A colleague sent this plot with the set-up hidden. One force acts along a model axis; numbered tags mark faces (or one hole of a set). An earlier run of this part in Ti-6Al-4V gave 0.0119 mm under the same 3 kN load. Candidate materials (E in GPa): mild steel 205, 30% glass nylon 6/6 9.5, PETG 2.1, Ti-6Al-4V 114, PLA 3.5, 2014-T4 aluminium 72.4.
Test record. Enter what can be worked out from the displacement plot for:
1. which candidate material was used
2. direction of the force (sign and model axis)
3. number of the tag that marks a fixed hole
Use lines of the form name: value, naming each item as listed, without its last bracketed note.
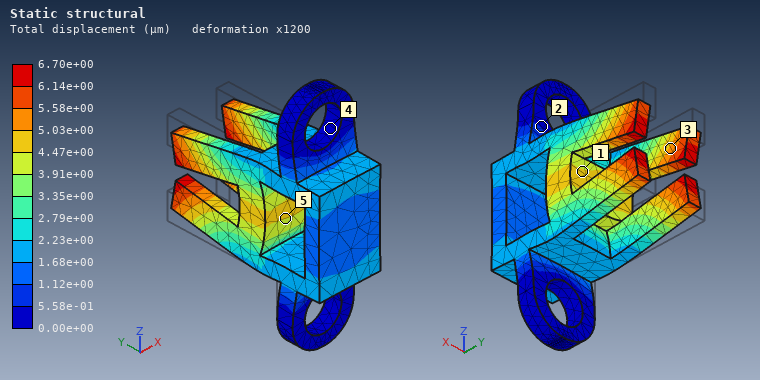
which candidate material was used: mild steel
direction of the force: -Y
number of the tag that marks a fixed hole: 4
